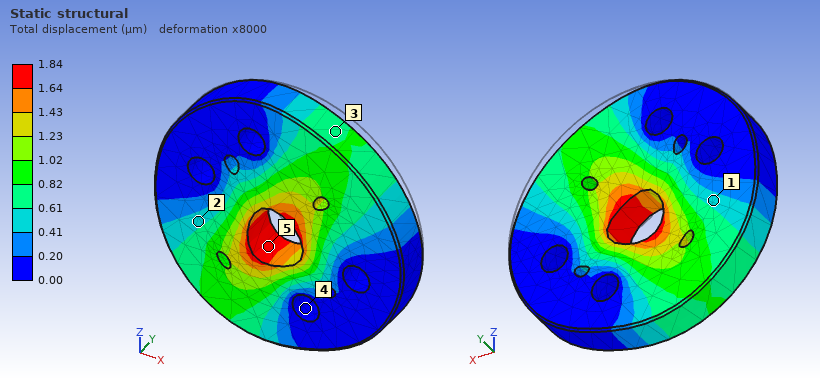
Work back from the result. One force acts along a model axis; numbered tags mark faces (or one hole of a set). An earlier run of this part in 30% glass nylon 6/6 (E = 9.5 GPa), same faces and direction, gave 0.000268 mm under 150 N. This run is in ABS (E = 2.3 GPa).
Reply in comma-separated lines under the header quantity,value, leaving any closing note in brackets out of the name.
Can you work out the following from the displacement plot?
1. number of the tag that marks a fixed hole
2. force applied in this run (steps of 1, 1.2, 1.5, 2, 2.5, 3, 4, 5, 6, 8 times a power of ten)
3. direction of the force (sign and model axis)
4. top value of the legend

quantity,value
number of the tag that marks a fixed hole,4
force applied in this run,250 N
direction of the force,-Z
top value of the legend,1.84 µm
